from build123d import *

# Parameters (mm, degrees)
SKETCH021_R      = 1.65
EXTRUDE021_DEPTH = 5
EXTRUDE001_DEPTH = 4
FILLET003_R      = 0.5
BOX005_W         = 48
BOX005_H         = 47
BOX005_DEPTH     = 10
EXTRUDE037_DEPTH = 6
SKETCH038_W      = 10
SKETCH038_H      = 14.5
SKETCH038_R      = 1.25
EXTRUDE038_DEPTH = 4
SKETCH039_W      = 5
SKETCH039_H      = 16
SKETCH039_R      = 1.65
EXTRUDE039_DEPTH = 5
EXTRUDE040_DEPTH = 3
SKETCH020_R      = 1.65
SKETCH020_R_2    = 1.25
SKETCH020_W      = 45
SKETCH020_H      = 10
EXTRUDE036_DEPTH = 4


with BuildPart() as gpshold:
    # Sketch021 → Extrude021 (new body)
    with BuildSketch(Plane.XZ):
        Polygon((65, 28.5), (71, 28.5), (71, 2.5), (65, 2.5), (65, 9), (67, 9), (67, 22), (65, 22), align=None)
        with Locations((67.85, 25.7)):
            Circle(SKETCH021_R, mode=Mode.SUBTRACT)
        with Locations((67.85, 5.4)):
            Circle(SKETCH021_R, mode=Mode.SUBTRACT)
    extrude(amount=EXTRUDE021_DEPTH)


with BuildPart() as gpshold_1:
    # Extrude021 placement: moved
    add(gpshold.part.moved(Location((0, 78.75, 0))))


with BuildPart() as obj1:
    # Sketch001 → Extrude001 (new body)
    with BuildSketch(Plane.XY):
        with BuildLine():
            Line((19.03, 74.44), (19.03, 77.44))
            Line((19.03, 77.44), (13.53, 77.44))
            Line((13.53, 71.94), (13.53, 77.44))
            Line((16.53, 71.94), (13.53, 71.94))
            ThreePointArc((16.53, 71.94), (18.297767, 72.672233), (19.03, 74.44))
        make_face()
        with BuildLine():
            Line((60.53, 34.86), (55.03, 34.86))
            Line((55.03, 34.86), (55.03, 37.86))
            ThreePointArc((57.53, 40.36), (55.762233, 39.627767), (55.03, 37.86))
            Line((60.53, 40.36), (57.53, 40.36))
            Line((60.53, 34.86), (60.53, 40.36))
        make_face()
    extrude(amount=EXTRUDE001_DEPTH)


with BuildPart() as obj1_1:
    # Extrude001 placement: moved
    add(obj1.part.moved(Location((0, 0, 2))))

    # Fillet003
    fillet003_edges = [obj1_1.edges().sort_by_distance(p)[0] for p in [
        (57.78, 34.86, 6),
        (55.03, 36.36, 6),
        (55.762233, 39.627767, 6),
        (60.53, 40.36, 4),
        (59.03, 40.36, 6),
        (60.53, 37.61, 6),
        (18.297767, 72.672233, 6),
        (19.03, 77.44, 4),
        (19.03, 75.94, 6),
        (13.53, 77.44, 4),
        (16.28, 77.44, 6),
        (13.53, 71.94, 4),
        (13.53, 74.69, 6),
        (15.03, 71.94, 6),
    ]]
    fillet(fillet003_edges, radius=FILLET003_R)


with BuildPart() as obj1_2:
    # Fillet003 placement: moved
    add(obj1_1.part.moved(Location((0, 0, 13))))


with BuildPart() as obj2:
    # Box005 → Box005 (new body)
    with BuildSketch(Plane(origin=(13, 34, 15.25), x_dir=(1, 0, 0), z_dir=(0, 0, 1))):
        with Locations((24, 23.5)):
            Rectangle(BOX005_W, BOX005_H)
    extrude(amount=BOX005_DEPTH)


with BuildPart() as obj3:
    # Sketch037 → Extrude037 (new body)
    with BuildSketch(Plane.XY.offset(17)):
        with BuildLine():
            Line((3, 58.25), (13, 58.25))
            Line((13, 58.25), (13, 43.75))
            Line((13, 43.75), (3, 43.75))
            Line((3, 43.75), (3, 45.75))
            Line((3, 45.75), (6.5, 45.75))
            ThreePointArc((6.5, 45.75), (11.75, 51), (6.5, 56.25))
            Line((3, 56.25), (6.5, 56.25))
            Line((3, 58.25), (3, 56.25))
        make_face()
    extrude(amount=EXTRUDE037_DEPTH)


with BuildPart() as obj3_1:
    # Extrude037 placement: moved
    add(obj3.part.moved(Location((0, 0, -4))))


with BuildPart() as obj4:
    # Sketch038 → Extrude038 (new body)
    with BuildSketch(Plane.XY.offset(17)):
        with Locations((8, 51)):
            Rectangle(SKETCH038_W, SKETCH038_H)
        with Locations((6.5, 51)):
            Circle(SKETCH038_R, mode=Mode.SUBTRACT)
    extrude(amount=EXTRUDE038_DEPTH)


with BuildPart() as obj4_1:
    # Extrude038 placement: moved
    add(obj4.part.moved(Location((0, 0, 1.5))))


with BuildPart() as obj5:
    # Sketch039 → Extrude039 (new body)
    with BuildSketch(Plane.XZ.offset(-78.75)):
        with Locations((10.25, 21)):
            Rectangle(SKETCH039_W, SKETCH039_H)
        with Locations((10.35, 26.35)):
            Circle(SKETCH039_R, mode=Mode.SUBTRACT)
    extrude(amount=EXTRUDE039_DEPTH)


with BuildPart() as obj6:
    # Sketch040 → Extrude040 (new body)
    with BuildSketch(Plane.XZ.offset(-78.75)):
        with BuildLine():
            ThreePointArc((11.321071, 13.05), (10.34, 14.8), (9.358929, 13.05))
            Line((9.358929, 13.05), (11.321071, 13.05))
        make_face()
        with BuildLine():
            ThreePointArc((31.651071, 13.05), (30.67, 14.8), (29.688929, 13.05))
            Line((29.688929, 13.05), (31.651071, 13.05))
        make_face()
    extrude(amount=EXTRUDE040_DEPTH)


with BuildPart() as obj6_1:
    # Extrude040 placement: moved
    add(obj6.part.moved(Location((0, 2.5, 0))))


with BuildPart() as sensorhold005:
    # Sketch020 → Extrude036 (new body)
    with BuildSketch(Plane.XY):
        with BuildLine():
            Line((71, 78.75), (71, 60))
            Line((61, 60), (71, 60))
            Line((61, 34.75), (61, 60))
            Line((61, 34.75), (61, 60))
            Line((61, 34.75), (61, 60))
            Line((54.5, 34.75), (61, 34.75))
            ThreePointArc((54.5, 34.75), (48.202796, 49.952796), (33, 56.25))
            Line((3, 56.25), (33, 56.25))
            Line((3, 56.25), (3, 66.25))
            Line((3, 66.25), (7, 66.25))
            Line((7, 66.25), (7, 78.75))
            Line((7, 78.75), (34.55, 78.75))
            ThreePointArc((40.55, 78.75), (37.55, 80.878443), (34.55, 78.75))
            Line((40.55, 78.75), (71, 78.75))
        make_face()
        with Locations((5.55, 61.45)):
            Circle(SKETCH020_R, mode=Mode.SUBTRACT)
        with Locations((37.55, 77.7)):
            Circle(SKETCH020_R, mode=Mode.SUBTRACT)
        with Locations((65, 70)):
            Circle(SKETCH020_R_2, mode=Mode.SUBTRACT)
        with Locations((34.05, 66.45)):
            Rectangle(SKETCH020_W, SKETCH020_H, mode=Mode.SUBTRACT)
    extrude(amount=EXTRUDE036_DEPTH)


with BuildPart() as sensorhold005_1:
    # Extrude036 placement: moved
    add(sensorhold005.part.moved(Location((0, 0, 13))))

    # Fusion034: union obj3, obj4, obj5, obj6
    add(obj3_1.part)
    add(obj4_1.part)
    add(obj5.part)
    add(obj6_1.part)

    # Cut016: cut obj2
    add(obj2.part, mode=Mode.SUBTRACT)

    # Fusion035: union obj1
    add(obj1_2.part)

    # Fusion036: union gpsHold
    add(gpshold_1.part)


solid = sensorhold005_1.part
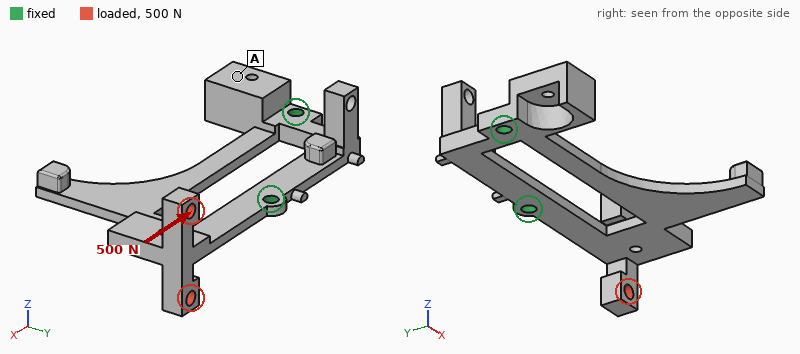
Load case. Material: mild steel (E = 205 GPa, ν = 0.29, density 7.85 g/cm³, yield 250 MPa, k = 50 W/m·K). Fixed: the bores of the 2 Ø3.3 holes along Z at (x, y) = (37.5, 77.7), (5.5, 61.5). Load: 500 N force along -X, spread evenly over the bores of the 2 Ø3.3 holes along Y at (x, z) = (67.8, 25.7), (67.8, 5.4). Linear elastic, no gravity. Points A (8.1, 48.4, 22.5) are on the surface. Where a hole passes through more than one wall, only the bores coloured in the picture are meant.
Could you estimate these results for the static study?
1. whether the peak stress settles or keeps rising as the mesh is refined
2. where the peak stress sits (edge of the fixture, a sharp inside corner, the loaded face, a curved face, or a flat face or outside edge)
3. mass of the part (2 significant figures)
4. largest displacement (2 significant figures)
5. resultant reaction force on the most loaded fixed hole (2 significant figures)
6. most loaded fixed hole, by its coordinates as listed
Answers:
keeps rising
edge of the fixture
40 g
0.20 mm
510 N
(37.5, 77.7)
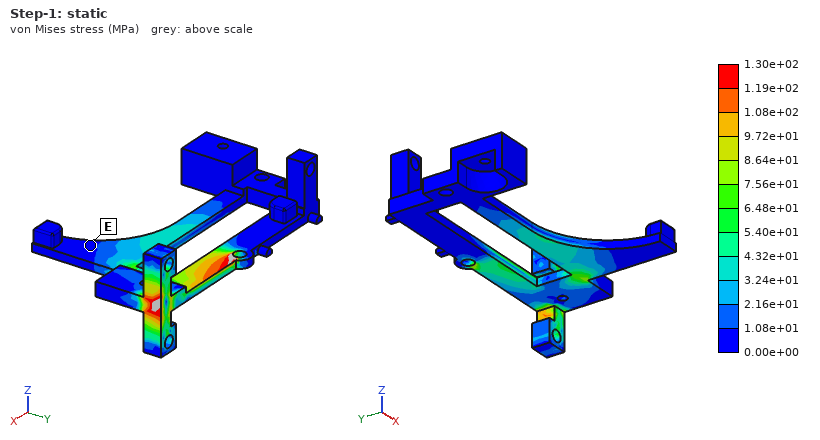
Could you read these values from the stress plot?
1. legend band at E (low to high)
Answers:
0.00e+00 to 1.08e+01 MPa
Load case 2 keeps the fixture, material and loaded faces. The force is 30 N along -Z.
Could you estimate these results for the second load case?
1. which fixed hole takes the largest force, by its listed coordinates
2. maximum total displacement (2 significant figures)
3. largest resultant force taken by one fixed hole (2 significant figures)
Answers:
(37.5, 77.7)
0.16 mm
36 N
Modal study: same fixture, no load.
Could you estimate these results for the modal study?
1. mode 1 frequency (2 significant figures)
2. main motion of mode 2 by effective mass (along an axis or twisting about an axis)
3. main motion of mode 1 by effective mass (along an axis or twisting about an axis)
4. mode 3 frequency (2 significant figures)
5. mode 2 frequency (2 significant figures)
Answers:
590 Hz
twisting about X
along Z
3400 Hz
1100 Hz
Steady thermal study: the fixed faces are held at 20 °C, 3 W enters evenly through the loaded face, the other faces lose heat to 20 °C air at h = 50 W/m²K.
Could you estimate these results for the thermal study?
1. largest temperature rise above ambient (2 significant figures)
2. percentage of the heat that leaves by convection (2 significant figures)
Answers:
39 K
75 %
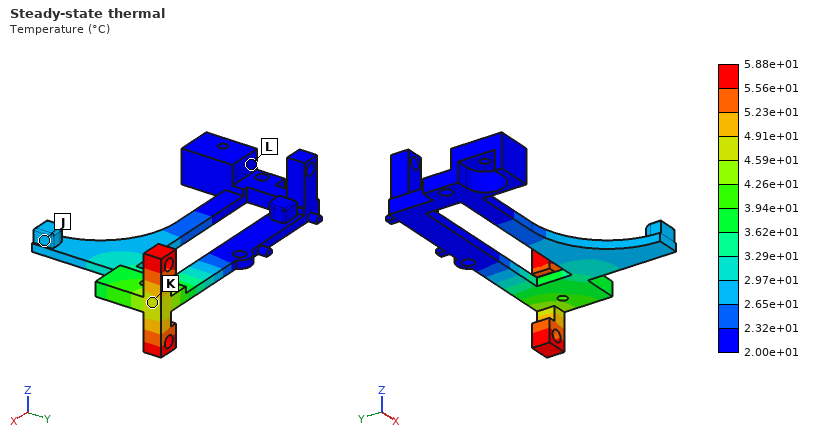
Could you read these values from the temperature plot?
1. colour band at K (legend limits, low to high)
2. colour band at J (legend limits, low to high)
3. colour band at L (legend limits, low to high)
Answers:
4.59e+01 to 4.91e+01 °C
2.65e+01 to 2.97e+01 °C
2.00e+01 to 2.32e+01 °C
